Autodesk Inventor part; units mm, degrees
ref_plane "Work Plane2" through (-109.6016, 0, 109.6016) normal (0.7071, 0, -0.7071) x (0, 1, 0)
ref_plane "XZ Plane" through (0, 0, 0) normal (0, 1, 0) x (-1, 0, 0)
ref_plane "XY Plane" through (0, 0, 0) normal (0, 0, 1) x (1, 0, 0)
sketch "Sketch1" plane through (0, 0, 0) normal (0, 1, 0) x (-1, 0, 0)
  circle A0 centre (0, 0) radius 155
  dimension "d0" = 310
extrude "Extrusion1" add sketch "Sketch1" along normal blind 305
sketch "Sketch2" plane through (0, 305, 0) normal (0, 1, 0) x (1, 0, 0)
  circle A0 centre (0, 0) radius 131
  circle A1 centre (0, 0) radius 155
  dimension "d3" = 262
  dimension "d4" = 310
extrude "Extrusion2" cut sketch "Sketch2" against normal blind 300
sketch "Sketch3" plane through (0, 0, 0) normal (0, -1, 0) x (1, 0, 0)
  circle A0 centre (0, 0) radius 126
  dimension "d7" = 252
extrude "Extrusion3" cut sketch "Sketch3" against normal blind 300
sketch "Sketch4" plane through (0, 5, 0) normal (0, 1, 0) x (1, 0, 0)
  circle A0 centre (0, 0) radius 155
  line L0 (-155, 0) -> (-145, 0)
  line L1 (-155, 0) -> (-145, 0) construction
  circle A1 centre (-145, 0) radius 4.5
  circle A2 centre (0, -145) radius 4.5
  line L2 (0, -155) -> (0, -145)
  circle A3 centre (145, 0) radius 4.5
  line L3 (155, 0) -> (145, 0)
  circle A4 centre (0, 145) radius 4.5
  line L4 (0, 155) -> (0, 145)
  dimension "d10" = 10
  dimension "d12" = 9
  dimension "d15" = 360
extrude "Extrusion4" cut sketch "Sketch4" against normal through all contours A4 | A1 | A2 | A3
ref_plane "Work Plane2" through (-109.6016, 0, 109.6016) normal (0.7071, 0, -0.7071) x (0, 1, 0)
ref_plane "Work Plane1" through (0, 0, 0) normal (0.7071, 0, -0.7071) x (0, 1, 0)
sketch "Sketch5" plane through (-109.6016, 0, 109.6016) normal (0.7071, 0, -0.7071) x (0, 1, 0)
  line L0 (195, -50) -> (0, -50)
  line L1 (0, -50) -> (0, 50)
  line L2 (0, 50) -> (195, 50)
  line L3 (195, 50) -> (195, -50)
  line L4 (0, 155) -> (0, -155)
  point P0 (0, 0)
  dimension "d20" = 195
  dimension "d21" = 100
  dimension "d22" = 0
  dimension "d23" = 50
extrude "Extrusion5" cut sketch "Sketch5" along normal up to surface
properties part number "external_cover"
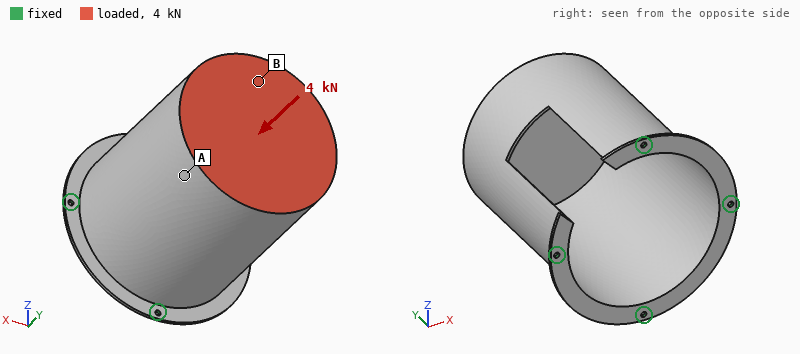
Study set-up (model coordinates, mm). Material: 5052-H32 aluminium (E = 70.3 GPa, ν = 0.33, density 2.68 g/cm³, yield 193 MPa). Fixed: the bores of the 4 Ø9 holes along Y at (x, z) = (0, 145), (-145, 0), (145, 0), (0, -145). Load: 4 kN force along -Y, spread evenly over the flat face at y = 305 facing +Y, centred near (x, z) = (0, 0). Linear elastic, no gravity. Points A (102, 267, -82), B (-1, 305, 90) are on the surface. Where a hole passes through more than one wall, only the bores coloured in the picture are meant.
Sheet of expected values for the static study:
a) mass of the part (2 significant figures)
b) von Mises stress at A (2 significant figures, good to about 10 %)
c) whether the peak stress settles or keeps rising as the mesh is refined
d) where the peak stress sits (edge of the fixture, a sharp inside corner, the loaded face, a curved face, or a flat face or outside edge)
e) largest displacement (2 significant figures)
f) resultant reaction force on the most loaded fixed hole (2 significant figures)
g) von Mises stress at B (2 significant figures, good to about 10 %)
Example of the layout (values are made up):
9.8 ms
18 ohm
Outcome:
4.0 kg
4.0 MPa
keeps rising
edge of the fixture
0.49 mm
1.0 kN
11 MPa
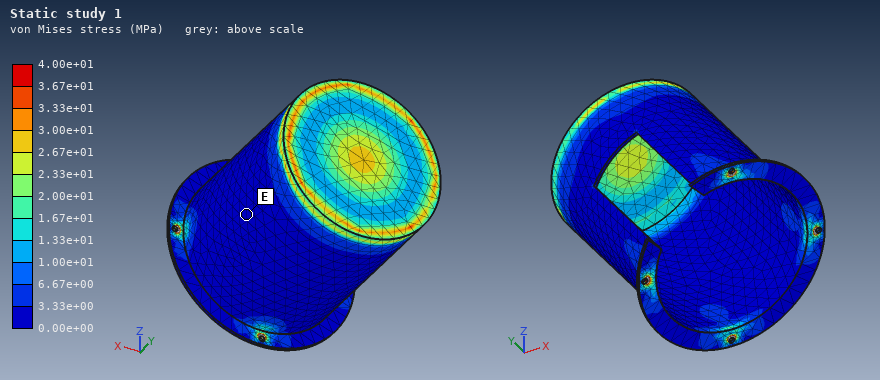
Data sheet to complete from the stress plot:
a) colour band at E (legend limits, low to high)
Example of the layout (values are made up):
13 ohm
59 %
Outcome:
0.00e+00 to 3.33e+00 MPa
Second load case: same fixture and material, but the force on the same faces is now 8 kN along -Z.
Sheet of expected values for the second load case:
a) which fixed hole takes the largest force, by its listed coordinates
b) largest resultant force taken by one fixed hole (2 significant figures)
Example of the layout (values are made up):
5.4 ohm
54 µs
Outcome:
(0, -145)
11 kN
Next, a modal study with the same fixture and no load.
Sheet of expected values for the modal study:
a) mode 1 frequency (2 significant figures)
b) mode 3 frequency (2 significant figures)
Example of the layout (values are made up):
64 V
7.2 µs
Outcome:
290 Hz
630 Hz
